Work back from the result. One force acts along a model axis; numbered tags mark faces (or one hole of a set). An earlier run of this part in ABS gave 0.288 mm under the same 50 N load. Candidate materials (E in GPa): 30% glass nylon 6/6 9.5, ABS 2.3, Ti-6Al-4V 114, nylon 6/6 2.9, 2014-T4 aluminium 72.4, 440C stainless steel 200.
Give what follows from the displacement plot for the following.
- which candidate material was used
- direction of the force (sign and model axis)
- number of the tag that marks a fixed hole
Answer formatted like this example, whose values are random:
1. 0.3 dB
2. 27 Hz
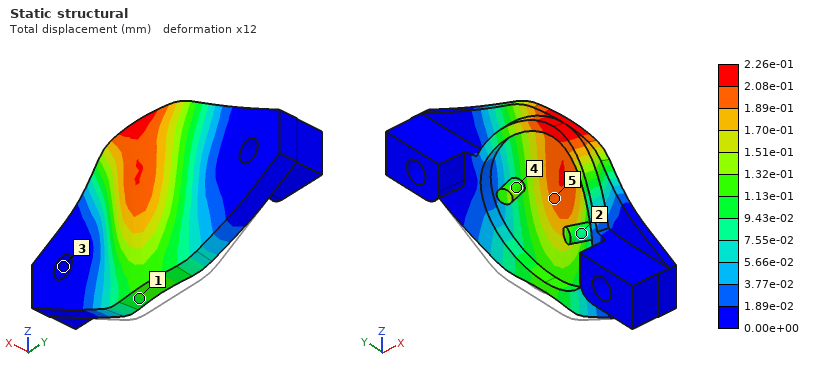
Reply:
1. nylon 6/6
2. +X
3. 3
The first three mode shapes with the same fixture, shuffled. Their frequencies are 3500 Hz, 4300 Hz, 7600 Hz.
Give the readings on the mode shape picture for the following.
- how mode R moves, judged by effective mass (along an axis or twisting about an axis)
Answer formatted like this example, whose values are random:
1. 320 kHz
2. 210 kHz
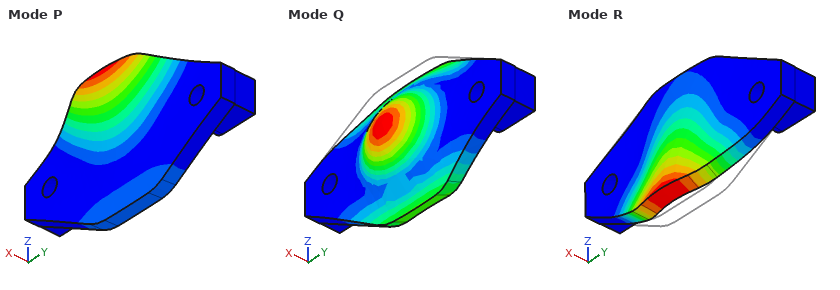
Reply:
1. along X
